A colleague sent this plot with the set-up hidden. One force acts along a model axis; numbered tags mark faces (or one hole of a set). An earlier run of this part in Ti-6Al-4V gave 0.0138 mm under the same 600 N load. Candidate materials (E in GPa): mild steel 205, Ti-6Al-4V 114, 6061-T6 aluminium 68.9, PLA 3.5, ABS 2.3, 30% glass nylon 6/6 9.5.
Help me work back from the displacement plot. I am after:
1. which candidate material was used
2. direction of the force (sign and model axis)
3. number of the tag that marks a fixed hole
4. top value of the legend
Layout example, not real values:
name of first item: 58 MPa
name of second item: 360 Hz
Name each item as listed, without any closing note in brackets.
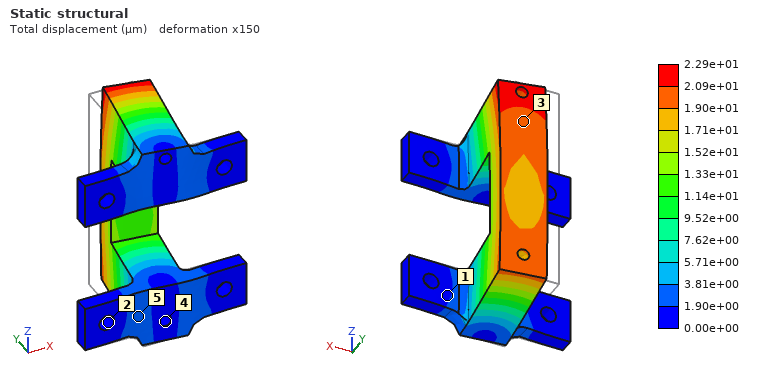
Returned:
which candidate material was used: 6061-T6 aluminium
direction of the force: +X
number of the tag that marks a fixed hole: 2
top value of the legend: 2.29e+01 µm
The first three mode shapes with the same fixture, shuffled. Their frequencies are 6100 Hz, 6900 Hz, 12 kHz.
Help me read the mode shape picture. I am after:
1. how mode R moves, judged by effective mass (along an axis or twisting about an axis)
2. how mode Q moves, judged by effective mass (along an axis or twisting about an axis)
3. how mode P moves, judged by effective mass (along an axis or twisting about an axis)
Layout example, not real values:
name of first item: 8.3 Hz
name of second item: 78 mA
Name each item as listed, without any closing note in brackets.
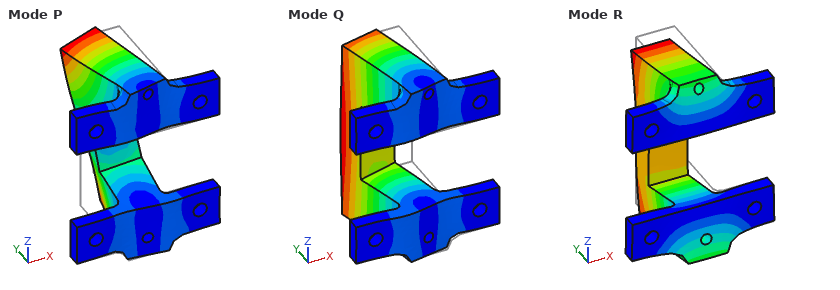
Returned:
how mode R moves, judged by effective mass: along Z
how mode Q moves, judged by effective mass: along X
how mode P moves, judged by effective mass: twisting about Y
